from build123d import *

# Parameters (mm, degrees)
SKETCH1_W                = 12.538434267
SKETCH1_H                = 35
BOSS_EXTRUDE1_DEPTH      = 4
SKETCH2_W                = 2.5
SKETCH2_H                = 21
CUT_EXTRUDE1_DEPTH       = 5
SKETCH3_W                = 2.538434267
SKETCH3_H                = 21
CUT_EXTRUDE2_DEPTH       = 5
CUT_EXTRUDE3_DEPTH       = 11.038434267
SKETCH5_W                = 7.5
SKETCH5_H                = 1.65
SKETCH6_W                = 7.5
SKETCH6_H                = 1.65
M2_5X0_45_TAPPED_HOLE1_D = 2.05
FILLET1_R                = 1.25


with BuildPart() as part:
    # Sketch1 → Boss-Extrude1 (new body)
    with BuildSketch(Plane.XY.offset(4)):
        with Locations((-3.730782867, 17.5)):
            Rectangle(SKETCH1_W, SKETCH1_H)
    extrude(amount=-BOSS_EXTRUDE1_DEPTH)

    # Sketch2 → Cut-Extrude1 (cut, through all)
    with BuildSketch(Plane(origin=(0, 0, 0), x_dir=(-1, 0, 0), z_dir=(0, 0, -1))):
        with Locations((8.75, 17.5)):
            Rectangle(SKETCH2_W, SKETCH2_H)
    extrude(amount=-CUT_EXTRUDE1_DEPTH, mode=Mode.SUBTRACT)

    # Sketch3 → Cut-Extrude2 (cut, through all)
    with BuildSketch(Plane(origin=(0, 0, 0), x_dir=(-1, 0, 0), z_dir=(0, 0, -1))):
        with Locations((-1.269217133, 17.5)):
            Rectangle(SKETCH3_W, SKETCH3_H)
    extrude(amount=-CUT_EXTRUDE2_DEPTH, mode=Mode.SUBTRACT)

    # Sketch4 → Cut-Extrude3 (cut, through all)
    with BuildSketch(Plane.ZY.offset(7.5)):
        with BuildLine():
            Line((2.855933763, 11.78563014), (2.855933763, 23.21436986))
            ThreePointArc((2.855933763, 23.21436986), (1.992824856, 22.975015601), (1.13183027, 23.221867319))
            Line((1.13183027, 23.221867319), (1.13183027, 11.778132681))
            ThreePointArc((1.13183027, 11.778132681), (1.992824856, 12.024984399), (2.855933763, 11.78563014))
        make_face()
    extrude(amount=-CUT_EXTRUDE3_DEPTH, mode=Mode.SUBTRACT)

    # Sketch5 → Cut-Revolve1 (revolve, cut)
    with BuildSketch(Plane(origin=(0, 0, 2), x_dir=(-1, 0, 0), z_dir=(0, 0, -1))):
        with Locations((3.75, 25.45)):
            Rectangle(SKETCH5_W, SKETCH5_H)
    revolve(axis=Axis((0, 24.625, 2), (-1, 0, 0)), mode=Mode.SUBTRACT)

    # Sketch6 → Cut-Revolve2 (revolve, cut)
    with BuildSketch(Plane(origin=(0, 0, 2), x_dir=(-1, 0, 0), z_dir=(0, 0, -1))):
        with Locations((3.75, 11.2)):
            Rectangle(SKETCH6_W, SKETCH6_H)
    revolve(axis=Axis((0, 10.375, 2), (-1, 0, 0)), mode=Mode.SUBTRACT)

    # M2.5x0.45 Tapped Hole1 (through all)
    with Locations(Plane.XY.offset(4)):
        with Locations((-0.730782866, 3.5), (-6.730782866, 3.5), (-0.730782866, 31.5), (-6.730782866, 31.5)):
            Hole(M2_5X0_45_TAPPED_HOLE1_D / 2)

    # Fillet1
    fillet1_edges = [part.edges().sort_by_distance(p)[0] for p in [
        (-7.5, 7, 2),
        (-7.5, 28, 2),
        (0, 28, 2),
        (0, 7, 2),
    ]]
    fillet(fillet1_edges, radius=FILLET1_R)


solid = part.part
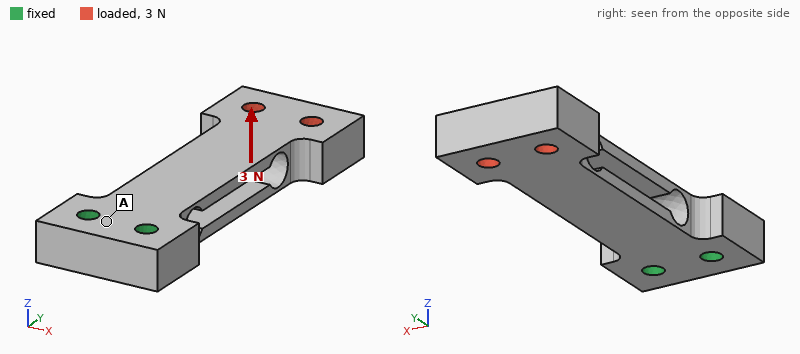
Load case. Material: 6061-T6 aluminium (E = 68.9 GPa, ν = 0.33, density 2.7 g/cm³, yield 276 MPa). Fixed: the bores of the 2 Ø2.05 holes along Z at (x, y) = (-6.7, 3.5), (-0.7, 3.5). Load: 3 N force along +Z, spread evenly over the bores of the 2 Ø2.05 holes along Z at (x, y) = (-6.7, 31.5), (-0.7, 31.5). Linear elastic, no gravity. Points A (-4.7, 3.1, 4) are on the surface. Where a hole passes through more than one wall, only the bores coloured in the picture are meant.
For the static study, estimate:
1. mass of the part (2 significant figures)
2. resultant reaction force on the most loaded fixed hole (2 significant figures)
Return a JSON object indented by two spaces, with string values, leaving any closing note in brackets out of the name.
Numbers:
{
  "mass of the part": "2.7 g",
  "resultant reaction force on the most loaded fixed hole": "1.5 N"
}
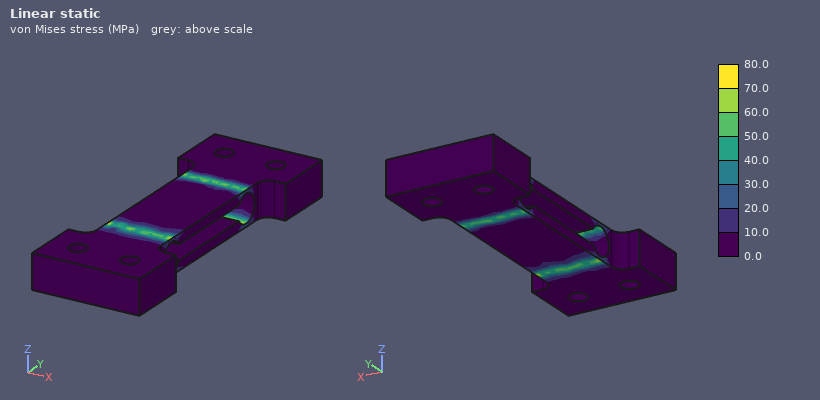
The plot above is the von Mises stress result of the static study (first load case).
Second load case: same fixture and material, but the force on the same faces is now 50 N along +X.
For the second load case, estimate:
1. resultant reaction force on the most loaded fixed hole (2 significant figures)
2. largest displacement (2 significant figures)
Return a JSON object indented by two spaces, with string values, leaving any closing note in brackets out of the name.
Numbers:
{
  "resultant reaction force on the most loaded fixed hole": "200 N",
  "largest displacement": "0.11 mm"
}
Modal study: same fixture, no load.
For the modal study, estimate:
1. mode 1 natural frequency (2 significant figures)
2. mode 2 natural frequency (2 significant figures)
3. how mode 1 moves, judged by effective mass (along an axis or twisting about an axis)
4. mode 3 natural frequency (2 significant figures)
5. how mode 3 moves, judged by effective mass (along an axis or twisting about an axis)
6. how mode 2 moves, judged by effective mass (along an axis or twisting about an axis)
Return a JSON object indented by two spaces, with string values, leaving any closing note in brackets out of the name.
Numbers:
{
  "mode 1 natural frequency": "760 Hz",
  "mode 2 natural frequency": "3700 Hz",
  "how mode 1 moves, judged by effective mass": "along Z",
  "mode 3 natural frequency": "4600 Hz",
  "how mode 3 moves, judged by effective mass": "twisting about Y",
  "how mode 2 moves, judged by effective mass": "along X"
}
